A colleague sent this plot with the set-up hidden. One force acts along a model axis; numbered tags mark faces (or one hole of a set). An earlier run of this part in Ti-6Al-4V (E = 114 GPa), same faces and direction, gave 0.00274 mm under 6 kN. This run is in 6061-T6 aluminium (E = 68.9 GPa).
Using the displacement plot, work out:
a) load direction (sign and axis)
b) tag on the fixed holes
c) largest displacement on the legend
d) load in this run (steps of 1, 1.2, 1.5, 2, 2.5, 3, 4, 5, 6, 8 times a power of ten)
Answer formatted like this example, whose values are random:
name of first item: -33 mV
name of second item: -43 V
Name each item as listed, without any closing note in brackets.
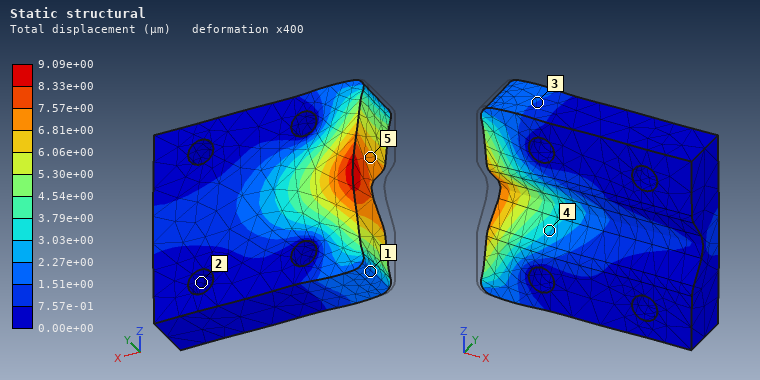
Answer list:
load direction: +X
tag on the fixed holes: 2
largest displacement on the legend: 9.09e+00 µm
load in this run: 12 kN
